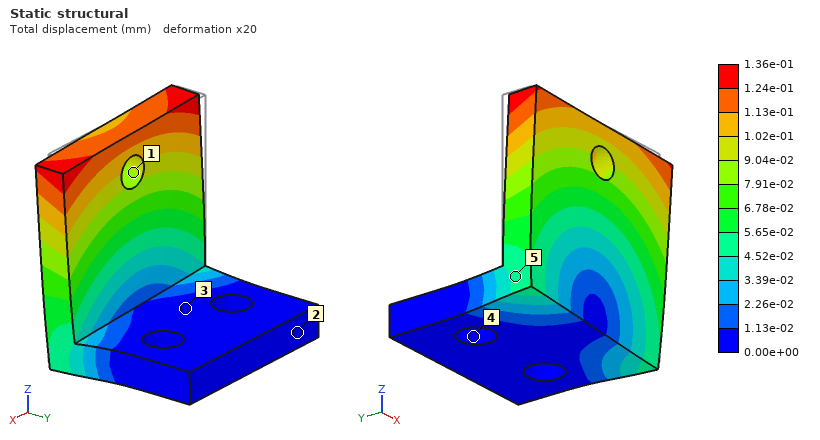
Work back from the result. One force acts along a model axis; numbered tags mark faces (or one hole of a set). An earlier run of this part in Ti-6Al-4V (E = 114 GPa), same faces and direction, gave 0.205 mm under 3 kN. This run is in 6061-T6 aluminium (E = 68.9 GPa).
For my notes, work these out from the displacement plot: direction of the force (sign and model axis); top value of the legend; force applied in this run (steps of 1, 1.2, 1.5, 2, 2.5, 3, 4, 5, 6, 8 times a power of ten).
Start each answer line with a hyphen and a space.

- +X
- 1.36e-01 mm
- 1.2 kN
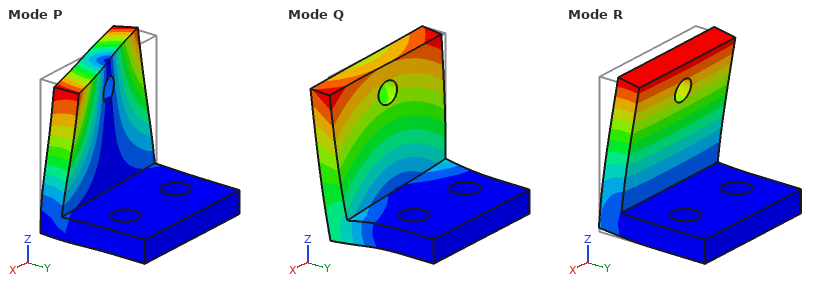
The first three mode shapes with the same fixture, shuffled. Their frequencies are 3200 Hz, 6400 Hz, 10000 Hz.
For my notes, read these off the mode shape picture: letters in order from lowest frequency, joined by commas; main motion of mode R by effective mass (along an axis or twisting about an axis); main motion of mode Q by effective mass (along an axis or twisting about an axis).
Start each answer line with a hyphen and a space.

- R, Q, P
- along Y
- along X
